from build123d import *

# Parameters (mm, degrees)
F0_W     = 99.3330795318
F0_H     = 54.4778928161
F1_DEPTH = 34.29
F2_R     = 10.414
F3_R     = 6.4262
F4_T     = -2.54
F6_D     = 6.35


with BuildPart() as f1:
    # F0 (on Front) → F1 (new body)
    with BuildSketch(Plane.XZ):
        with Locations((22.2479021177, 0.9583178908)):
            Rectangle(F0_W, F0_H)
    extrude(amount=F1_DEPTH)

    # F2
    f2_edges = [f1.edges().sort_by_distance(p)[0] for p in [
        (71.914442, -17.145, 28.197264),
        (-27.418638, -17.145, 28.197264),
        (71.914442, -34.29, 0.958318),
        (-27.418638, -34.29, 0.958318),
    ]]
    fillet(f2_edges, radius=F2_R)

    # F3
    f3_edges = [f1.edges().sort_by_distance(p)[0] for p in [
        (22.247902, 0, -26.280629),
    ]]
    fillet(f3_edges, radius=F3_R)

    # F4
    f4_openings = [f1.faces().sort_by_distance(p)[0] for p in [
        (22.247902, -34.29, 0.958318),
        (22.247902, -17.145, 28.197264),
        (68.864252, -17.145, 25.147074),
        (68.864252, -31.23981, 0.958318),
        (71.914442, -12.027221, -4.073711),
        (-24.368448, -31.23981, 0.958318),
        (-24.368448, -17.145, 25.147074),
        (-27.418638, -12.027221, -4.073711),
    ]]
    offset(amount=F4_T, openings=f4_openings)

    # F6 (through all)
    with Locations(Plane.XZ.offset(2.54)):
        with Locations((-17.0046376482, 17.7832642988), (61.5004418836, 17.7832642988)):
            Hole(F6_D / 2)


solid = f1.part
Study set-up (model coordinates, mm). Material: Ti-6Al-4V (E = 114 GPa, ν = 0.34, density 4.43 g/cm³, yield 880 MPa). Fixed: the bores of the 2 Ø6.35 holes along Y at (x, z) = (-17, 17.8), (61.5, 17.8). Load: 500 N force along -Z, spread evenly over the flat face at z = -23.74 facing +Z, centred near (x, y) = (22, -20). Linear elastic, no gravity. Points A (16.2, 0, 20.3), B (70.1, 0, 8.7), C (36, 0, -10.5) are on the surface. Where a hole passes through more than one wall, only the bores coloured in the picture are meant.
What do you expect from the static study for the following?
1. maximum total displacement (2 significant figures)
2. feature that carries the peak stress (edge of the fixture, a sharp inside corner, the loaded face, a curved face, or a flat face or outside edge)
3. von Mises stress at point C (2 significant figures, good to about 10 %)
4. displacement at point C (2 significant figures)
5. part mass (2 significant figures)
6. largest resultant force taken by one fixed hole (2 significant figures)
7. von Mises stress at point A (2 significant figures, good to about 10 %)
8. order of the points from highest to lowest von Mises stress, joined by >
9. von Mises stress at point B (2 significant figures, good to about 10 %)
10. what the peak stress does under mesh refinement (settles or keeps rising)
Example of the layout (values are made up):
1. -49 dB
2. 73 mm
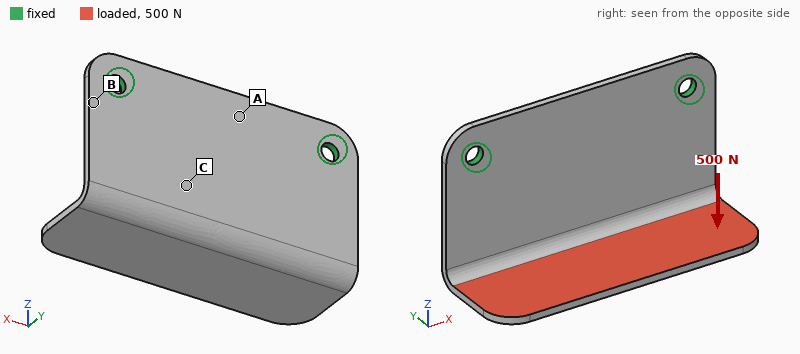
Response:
1. 1.2 mm
2. edge of the fixture
3. 75 MPa
4. 0.31 mm
5. 92 g
6. 270 N
7. 27 MPa
8. B > C > A
9. 120 MPa
10. keeps rising
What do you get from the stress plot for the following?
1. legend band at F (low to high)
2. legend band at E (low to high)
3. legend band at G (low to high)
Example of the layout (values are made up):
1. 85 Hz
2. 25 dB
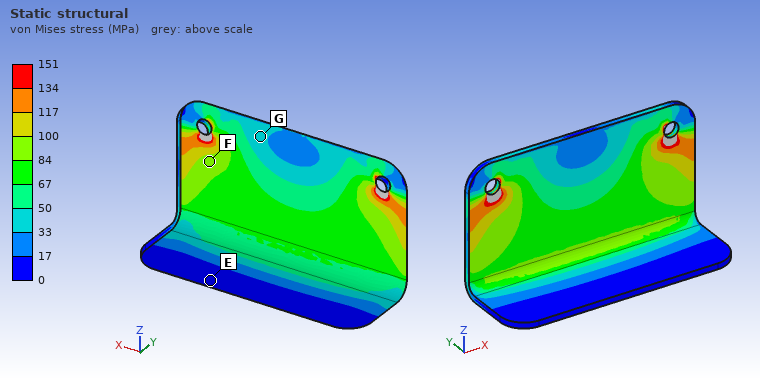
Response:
1. 84 to 100 MPa
2. 0 to 17 MPa
3. 33 to 50 MPa
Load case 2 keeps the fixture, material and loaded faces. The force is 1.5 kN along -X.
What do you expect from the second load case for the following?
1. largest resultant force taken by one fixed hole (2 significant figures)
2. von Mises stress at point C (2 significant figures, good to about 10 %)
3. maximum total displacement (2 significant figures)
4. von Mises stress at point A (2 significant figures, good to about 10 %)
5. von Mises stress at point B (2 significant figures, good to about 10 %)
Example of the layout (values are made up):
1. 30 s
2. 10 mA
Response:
1. 1.1 kN
2. 87 MPa
3. 1.1 mm
4. 26 MPa
5. 210 MPa
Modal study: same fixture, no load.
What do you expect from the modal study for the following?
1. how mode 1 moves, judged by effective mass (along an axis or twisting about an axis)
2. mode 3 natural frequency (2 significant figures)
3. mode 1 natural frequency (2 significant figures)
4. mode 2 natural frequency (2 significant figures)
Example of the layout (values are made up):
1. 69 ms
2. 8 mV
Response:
1. along Y
2. 1400 Hz
3. 450 Hz
4. 860 Hz
